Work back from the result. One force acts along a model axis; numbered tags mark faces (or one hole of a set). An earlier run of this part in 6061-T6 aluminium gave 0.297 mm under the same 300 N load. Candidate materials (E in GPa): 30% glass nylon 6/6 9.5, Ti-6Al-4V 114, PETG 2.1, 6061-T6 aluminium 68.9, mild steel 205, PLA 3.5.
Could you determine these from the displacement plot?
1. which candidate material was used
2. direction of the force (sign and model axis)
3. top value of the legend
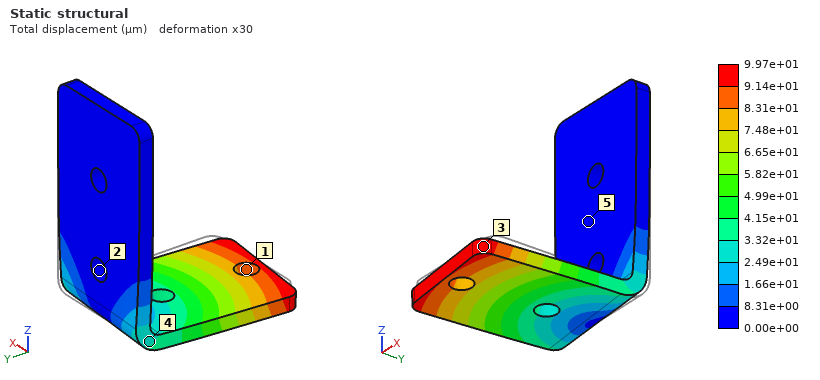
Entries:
mild steel
-X
9.97e+01 µm
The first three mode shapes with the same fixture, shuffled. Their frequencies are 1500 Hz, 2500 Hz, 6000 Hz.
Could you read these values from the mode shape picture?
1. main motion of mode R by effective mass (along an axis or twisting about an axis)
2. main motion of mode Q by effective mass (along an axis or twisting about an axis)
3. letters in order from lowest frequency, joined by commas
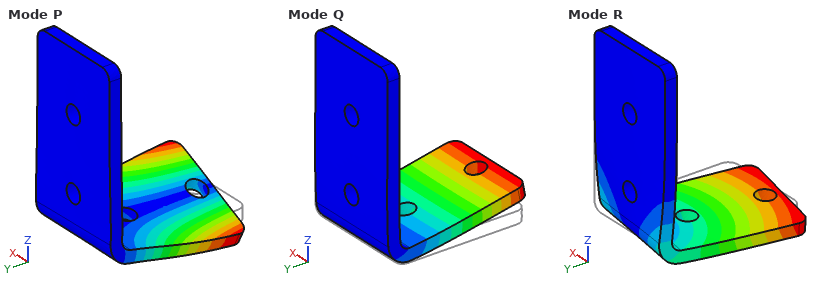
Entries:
along X
along Z
Q, R, P
